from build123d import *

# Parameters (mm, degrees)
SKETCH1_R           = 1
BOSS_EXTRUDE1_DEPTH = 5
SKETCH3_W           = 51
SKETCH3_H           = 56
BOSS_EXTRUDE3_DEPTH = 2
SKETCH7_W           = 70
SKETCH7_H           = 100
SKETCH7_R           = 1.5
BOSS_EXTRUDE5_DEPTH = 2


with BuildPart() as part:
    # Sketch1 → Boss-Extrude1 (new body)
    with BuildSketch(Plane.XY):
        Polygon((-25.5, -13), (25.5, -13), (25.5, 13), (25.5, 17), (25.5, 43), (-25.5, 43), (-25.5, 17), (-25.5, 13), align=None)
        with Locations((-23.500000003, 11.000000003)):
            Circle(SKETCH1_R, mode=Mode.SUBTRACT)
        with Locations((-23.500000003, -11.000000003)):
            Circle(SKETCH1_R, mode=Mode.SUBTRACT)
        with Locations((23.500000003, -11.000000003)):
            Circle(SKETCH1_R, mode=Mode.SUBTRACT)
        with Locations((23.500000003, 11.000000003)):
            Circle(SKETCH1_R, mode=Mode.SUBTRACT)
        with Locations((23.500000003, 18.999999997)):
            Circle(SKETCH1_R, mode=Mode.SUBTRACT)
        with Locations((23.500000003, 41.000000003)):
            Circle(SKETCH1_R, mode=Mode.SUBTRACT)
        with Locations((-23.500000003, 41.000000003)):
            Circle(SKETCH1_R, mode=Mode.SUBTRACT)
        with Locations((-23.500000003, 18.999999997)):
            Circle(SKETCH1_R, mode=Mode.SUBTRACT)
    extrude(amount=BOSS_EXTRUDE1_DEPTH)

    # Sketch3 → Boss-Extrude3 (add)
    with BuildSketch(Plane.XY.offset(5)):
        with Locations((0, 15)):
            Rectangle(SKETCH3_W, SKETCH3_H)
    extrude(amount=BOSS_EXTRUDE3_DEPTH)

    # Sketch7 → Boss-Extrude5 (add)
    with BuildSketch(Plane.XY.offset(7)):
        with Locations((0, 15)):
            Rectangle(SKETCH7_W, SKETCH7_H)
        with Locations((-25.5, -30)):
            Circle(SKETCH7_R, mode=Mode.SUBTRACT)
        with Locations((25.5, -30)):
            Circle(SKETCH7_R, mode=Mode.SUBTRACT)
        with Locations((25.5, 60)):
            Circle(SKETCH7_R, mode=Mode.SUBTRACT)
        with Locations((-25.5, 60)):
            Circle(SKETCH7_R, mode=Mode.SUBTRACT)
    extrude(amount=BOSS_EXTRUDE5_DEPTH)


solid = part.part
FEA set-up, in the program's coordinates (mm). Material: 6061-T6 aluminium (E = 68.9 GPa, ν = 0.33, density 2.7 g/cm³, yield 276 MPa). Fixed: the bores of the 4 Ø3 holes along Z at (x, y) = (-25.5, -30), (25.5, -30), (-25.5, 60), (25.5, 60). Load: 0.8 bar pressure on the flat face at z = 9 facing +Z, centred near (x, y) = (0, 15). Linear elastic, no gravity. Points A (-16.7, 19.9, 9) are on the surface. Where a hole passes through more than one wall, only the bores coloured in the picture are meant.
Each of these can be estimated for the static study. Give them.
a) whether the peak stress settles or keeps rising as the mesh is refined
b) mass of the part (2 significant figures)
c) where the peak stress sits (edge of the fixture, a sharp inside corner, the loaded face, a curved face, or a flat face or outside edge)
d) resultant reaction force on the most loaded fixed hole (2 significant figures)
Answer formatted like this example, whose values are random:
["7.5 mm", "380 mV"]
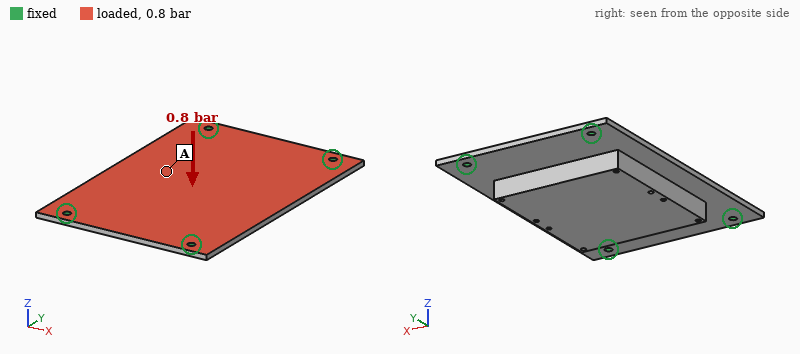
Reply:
["keeps rising", "91 g", "edge of the fixture", "170 N"]
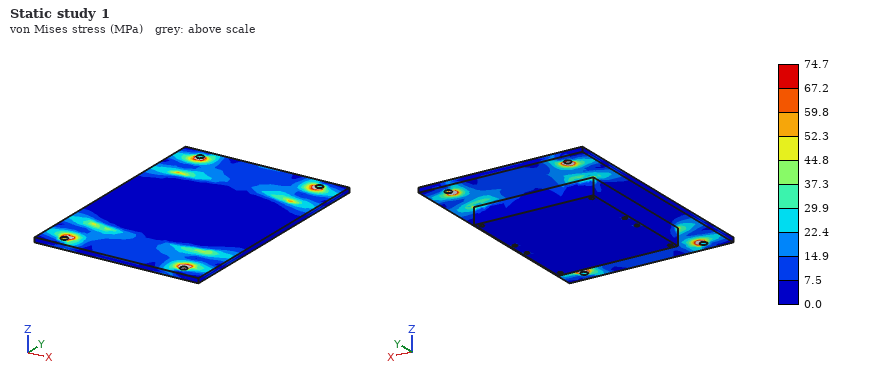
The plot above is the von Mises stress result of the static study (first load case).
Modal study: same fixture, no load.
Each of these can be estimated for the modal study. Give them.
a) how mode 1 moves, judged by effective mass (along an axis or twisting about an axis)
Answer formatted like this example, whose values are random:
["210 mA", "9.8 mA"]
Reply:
["along Z"]
